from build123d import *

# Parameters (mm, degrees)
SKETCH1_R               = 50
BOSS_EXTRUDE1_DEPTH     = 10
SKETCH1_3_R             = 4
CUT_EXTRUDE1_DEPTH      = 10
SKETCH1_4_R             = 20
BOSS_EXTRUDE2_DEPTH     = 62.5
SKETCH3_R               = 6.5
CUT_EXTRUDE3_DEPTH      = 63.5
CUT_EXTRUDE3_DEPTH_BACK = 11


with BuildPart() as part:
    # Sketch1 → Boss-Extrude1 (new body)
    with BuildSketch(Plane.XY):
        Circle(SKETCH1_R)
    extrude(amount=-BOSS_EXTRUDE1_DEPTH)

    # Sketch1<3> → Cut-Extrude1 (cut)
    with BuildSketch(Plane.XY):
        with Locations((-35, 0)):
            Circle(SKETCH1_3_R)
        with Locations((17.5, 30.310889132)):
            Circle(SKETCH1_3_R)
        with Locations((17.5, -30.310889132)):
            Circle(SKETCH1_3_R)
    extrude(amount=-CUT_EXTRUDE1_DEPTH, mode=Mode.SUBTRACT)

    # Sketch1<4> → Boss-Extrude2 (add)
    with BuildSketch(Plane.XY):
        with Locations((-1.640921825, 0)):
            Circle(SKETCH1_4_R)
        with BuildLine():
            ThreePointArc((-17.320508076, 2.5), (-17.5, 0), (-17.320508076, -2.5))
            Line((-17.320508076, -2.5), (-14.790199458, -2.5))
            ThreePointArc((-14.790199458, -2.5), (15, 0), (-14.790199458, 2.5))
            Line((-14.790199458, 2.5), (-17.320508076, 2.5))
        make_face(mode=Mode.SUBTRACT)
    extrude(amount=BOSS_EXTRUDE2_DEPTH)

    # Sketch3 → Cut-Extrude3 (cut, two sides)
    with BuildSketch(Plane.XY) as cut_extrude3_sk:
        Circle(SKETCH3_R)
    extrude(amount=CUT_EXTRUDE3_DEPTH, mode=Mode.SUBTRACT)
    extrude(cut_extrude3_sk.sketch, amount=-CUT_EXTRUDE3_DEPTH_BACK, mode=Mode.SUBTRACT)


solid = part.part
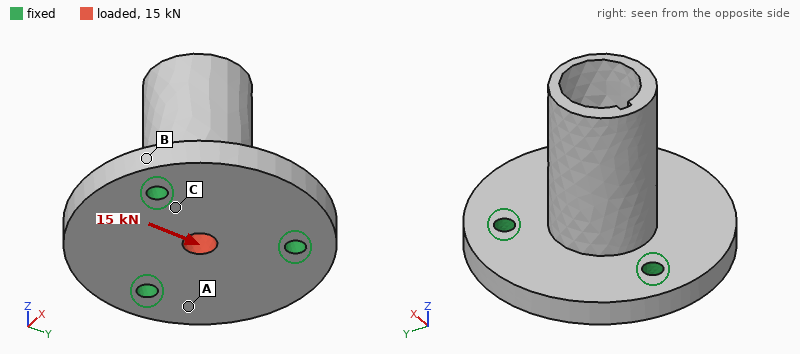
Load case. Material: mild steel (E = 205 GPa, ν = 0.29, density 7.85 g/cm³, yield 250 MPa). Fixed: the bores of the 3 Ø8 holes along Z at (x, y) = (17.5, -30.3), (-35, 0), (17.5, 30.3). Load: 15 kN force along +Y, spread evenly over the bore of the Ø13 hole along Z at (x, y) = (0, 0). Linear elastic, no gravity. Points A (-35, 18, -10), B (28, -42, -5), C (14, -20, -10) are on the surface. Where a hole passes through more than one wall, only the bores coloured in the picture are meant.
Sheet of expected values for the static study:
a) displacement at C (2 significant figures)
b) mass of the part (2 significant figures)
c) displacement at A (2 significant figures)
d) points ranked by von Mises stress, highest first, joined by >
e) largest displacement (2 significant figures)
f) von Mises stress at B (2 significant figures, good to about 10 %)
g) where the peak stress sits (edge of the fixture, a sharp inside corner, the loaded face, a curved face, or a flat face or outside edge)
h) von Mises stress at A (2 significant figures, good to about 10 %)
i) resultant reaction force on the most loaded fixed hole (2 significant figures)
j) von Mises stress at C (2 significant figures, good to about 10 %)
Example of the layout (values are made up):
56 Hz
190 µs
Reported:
1.2 µm
860 g
1.1 µm
C > A > B
4.9 µm
5.8 MPa
the loaded face
9.3 MPa
5.3 kN
28 MPa
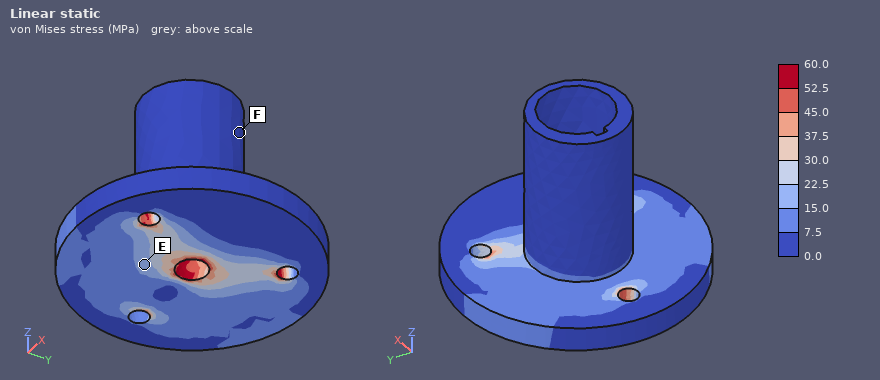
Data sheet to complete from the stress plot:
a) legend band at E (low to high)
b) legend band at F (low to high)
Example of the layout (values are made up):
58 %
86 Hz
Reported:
15.0 to 22.5 MPa
0.0 to 7.5 MPa
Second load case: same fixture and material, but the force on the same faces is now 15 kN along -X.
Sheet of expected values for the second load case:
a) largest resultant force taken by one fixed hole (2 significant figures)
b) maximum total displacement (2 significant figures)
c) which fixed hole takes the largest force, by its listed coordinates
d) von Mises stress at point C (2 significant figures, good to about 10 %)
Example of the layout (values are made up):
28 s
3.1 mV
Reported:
5.6 kN
5.0 µm
(-35, 0)
18 MPa
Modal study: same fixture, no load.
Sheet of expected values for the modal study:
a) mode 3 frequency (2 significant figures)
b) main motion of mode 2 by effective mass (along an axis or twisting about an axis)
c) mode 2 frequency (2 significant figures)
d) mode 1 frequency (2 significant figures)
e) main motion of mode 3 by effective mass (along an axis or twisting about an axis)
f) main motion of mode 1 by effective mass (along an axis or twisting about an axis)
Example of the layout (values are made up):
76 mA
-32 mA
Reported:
7800 Hz
along X
4300 Hz
4000 Hz
along Z
along Y
